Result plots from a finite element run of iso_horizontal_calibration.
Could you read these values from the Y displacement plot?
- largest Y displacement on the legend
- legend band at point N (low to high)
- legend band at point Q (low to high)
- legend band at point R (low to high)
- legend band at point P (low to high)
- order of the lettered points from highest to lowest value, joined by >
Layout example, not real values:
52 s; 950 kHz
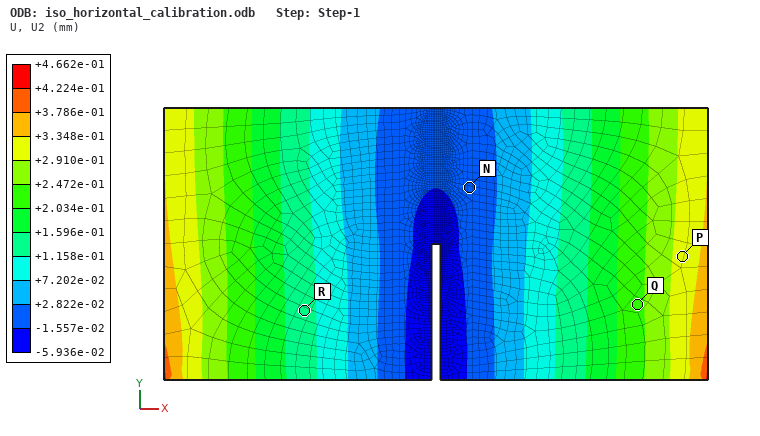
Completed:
+4.662e-01 mm; -1.557e-02 to +2.822e-02 mm; +2.034e-01 to +2.472e-01 mm; +1.158e-01 to +1.596e-01 mm; +2.910e-01 to +3.348e-01 mm; P > Q > R > N
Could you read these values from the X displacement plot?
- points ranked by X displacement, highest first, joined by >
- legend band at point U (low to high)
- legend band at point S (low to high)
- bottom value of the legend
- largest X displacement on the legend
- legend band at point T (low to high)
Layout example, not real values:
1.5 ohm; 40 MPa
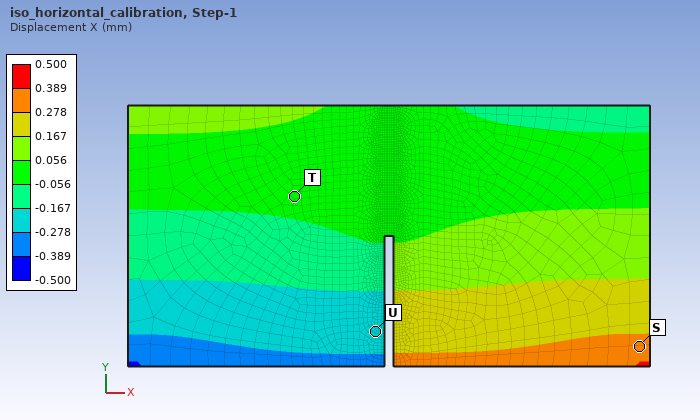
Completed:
S > T > U; -0.278 to -0.167 mm; 0.278 to 0.389 mm; -0.500 mm; 0.500 mm; -0.056 to 0.056 mm
